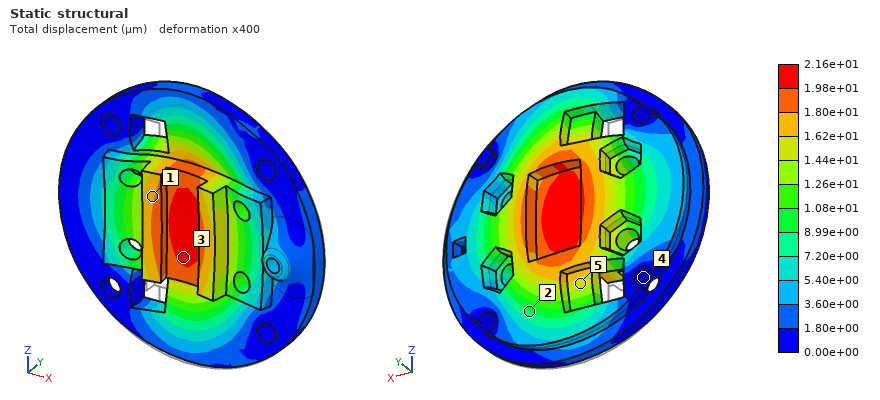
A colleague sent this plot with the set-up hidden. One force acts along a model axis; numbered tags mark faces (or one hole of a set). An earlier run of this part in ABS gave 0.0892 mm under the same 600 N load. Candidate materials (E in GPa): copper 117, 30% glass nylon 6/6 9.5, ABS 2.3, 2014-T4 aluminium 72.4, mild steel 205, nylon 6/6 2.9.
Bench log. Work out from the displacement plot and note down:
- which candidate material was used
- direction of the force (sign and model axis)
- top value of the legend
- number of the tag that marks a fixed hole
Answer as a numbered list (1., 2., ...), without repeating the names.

1. 30% glass nylon 6/6
2. +Y
3. 2.16e+01 µm
4. 4
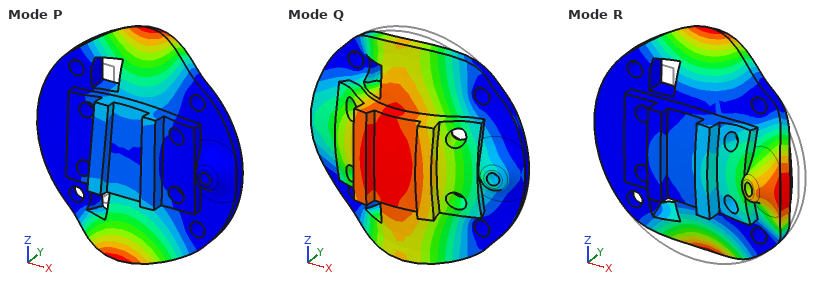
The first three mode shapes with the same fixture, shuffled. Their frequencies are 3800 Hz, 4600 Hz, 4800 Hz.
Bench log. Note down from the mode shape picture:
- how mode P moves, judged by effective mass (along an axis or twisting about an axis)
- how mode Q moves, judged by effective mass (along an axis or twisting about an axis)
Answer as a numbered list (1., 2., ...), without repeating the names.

1. twisting about X
2. along Y
